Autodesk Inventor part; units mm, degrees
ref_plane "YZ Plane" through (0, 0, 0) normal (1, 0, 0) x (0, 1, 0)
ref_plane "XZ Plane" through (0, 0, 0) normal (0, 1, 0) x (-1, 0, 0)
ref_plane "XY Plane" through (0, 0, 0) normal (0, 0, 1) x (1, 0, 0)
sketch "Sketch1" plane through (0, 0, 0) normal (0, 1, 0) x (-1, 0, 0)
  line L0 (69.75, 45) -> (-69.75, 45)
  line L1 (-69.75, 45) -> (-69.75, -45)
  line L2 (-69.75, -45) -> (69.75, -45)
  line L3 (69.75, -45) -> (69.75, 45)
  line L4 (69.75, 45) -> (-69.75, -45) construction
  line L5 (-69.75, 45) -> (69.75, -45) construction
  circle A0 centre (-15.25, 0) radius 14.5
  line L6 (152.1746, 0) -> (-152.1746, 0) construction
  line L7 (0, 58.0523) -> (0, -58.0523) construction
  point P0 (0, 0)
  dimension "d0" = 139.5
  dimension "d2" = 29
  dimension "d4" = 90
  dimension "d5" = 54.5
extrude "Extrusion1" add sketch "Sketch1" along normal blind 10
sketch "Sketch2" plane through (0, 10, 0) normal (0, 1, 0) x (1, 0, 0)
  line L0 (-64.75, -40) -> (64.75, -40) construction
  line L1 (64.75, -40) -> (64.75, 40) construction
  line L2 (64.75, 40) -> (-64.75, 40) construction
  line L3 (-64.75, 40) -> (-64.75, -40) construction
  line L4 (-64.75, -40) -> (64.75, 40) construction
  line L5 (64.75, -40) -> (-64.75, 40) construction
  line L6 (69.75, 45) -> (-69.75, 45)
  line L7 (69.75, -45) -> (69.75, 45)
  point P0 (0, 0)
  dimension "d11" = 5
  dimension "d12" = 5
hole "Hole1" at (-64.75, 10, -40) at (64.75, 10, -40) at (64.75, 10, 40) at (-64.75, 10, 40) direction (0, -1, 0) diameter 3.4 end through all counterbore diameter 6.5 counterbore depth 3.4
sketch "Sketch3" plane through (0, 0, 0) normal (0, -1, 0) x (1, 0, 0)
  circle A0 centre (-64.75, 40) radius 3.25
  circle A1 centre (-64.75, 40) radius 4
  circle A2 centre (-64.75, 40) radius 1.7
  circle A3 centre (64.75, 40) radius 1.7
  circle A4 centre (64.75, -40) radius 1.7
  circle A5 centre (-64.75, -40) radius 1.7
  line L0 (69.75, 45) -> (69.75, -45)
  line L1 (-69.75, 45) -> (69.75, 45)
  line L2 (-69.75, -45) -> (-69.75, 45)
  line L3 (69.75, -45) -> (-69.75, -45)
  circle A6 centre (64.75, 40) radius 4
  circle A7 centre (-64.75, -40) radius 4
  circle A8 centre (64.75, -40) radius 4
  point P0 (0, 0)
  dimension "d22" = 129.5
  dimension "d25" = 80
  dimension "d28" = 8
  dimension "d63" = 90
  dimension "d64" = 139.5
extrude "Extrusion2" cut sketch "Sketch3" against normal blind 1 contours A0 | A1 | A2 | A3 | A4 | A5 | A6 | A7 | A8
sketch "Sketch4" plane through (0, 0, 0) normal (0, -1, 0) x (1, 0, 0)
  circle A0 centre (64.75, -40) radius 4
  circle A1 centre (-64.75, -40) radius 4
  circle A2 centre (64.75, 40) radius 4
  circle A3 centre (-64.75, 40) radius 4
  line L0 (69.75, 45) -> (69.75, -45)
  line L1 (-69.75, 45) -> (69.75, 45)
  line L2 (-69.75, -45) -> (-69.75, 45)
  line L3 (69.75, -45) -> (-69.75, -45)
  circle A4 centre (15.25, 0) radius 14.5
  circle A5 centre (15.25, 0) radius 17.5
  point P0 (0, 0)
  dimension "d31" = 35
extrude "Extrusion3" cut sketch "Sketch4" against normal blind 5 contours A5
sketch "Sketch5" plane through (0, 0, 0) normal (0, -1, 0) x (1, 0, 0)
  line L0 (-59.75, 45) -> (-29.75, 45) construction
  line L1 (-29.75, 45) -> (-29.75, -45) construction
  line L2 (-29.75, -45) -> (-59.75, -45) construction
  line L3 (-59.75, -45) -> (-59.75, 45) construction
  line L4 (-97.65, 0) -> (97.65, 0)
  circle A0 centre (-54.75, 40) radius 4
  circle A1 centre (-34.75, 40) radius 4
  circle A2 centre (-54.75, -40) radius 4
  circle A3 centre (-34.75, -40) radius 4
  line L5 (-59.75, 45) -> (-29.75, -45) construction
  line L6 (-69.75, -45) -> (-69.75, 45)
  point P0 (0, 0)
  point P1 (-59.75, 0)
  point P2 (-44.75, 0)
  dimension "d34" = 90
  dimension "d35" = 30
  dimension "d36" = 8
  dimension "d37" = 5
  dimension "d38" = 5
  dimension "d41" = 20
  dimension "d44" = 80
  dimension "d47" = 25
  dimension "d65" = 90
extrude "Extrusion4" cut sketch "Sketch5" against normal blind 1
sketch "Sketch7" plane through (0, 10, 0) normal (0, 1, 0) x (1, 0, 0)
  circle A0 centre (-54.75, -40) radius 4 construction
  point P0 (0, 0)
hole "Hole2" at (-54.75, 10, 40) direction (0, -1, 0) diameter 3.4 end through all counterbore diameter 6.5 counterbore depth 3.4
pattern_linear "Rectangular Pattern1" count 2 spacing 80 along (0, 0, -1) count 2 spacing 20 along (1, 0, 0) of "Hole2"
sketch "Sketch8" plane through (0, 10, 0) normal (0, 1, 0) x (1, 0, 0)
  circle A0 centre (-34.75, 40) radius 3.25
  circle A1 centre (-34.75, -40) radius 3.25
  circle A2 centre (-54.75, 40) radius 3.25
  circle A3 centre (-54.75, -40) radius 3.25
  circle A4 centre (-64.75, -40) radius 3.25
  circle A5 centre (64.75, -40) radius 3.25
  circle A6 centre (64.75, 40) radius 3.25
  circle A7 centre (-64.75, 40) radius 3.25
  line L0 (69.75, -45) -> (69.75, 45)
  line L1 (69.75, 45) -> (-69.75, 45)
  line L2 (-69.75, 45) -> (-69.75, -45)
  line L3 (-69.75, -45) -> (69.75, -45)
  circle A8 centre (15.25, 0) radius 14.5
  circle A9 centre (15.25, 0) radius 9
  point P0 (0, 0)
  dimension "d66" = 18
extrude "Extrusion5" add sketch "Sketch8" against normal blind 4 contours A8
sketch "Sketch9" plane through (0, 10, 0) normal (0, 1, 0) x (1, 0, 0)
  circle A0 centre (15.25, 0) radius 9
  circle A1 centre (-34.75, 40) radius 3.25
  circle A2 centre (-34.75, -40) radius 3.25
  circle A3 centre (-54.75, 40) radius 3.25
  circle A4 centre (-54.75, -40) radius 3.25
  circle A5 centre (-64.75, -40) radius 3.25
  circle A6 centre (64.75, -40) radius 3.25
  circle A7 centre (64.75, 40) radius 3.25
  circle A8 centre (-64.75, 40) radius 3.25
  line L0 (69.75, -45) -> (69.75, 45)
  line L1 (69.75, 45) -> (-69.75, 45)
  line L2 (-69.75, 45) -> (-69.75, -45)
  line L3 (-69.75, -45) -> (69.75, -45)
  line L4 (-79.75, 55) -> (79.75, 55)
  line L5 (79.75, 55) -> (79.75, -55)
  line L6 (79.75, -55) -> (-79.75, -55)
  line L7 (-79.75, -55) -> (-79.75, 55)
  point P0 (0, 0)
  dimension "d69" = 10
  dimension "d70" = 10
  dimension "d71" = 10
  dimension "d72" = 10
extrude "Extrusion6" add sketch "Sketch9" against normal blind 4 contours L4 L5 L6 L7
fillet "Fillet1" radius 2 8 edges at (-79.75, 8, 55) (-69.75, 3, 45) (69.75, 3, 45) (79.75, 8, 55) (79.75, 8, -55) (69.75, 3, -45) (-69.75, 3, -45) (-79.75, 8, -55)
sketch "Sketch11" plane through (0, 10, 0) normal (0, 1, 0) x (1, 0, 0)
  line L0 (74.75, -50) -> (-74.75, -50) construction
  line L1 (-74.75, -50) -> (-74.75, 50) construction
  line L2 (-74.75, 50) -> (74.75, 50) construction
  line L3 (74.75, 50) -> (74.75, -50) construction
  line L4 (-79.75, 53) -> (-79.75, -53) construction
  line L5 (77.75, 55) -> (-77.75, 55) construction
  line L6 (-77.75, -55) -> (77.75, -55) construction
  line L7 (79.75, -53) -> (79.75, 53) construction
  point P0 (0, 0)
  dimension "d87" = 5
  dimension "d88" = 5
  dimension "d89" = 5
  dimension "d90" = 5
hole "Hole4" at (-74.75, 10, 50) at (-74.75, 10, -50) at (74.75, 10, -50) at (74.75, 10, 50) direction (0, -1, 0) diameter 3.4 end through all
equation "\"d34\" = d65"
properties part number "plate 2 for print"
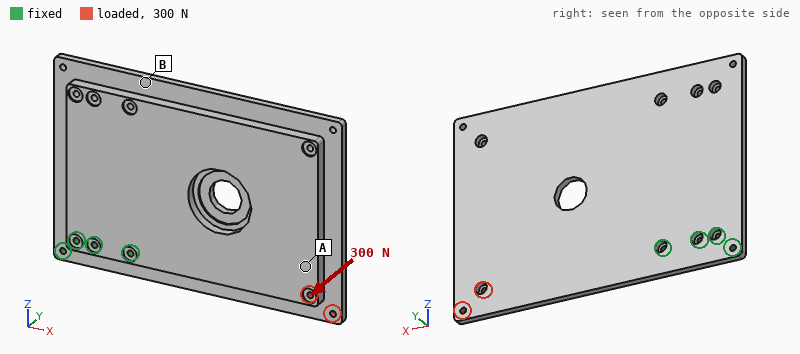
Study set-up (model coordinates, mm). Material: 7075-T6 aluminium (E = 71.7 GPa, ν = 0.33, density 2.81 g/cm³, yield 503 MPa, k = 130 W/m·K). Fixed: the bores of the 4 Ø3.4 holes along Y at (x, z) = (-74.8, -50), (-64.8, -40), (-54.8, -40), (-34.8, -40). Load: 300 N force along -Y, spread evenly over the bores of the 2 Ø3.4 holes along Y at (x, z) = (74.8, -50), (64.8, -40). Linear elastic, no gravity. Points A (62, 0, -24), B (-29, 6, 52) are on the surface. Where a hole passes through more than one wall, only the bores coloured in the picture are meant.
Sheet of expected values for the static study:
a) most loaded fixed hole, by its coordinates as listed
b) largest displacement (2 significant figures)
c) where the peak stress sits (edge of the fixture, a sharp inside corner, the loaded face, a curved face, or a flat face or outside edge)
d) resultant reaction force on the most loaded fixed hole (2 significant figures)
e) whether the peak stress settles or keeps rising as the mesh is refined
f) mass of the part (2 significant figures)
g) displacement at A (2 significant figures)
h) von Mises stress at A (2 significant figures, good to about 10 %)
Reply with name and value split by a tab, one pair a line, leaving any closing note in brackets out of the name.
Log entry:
most loaded fixed hole, by its coordinates as listed	(-34.8, -40)
largest displacement	0.54 mm
where the peak stress sits	edge of the fixture
resultant reaction force on the most loaded fixed hole	1.4 kN
whether the peak stress settles or keeps rising as the mesh is refined	keeps rising
mass of the part	390 g
displacement at A	0.39 mm
von Mises stress at A	11 MPa
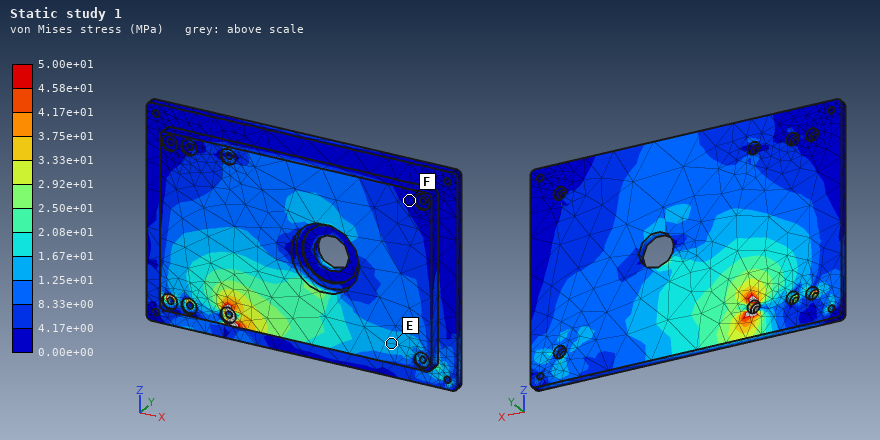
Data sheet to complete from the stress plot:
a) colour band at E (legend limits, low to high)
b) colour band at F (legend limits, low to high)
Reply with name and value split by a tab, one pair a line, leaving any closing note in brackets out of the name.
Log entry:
colour band at E	1.25e+01 to 1.67e+01 MPa
colour band at F	0.00e+00 to 4.17e+00 MPa
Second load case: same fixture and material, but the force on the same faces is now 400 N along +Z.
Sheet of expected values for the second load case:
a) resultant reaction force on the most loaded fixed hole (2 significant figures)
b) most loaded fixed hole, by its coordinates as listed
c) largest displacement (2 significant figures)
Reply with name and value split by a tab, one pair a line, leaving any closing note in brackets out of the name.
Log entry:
resultant reaction force on the most loaded fixed hole	1.6 kN
most loaded fixed hole, by its coordinates as listed	(-34.8, -40)
largest displacement	48 µm
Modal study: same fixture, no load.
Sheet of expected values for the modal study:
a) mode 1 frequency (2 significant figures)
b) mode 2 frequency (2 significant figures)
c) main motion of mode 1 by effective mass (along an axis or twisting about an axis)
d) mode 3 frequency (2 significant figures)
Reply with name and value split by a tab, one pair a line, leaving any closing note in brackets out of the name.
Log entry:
mode 1 frequency	360 Hz
mode 2 frequency	700 Hz
main motion of mode 1 by effective mass	along Y
mode 3 frequency	1400 Hz
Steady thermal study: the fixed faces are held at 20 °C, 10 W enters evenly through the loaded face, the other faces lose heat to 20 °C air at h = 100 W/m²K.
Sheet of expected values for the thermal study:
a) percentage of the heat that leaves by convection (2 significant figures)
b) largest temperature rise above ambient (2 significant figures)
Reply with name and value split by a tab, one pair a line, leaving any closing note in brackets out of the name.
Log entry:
percentage of the heat that leaves by convection	81 %
largest temperature rise above ambient	15 K
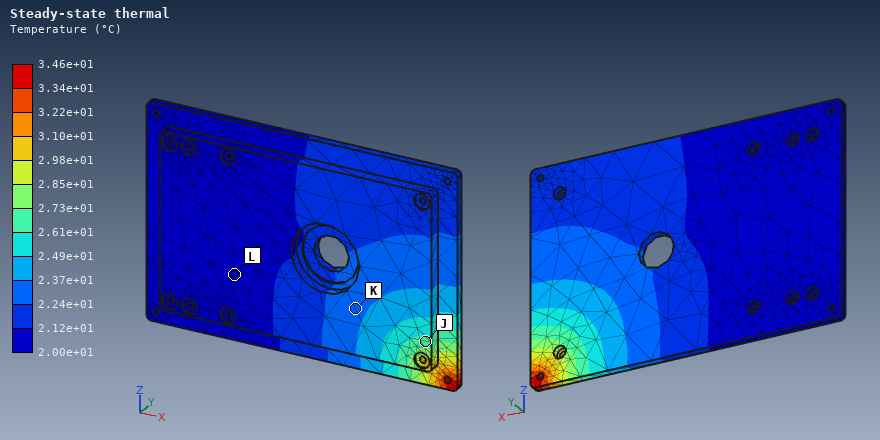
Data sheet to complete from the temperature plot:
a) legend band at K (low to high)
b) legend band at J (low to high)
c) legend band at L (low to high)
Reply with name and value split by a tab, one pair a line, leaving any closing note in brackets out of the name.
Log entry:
legend band at K	2.24e+01 to 2.37e+01 °C
legend band at J	2.61e+01 to 2.73e+01 °C
legend band at L	2.00e+01 to 2.12e+01 °C
